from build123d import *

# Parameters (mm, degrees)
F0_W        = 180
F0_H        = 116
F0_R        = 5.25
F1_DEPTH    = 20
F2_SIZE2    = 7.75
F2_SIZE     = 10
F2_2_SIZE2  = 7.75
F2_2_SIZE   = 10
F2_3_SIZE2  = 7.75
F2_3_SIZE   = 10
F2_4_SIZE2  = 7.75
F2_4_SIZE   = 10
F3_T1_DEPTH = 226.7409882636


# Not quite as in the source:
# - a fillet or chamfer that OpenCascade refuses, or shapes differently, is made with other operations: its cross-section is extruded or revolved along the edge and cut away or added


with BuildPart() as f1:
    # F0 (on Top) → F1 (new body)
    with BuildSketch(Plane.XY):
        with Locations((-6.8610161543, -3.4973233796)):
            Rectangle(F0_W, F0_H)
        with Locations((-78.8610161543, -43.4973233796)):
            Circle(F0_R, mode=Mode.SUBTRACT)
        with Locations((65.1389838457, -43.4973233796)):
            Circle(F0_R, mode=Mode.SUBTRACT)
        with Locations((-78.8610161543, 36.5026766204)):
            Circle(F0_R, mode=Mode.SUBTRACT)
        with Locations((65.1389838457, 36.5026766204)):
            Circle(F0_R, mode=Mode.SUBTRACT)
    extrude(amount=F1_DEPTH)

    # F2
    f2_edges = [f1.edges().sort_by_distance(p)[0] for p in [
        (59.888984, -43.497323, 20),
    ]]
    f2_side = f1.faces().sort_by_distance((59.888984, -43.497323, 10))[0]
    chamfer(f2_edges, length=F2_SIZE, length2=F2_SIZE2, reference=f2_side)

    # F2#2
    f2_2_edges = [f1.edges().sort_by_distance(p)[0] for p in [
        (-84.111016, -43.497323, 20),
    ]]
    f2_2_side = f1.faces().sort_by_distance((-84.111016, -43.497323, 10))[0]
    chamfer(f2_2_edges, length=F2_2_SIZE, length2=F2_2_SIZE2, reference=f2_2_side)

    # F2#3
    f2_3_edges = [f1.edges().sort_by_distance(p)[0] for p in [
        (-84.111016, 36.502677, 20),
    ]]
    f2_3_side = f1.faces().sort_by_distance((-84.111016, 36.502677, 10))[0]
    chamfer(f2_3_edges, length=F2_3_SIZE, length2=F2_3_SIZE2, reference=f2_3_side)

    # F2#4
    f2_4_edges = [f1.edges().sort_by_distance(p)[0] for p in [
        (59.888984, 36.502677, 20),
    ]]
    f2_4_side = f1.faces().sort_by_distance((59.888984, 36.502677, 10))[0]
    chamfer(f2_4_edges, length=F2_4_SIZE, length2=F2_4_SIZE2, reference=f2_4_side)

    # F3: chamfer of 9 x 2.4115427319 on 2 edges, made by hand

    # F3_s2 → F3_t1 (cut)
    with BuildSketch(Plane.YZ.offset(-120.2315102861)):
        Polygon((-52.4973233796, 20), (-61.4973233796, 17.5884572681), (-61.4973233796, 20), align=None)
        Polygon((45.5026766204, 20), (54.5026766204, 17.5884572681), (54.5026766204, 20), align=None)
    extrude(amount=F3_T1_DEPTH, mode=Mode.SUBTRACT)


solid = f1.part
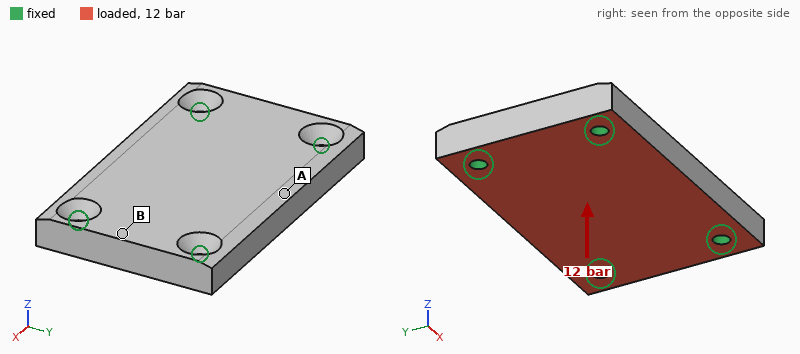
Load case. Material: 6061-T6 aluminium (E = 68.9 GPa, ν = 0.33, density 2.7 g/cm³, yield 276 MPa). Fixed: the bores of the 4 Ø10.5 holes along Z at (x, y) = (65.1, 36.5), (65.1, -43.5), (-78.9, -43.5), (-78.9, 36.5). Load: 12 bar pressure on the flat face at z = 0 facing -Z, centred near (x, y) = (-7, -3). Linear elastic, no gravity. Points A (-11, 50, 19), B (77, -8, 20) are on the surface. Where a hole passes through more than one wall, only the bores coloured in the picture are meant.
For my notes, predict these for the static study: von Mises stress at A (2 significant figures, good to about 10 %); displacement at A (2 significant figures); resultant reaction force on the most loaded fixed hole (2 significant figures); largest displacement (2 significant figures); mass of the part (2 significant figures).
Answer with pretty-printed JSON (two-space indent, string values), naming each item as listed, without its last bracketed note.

{
  "von Mises stress at A": "26 MPa",
  "displacement at A": "67 µm",
  "resultant reaction force on the most loaded fixed hole": "7.1 kN",
  "largest displacement": "69 µm",
  "mass of the part": "1.1 kg"
}
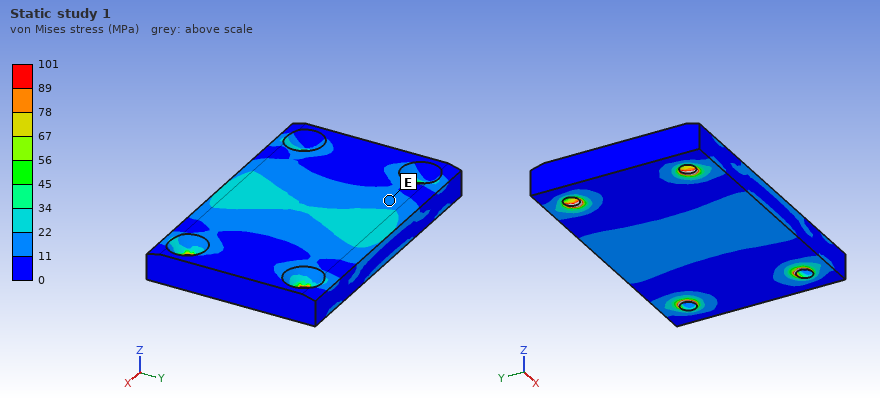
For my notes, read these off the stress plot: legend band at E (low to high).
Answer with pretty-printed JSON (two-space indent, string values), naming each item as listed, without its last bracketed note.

{
  "legend band at E": "11 to 22 MPa"
}
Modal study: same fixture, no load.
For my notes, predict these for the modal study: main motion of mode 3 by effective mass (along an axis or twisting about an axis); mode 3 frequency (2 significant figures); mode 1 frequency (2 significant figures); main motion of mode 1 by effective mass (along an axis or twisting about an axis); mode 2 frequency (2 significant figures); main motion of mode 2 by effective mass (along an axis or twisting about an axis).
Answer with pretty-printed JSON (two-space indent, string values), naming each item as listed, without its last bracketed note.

{
  "main motion of mode 3 by effective mass": "along Y",
  "mode 3 frequency": "8200 Hz",
  "mode 1 frequency": "3300 Hz",
  "main motion of mode 1 by effective mass": "along Z",
  "mode 2 frequency": "4800 Hz",
  "main motion of mode 2 by effective mass": "twisting about X"
}
